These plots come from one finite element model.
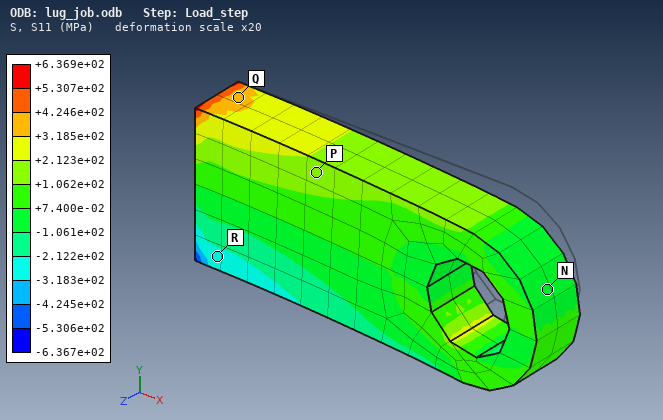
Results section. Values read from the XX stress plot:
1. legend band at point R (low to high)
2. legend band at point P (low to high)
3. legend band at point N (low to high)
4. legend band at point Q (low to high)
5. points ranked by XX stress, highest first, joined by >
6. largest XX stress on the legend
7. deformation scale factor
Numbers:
-3.183e+02 to -2.122e+02 MPa
+1.062e+02 to +2.123e+02 MPa
-1.061e+02 to +7.400e-02 MPa
+3.185e+02 to +4.246e+02 MPa
Q > P > N > R
+6.369e+02 MPa
20
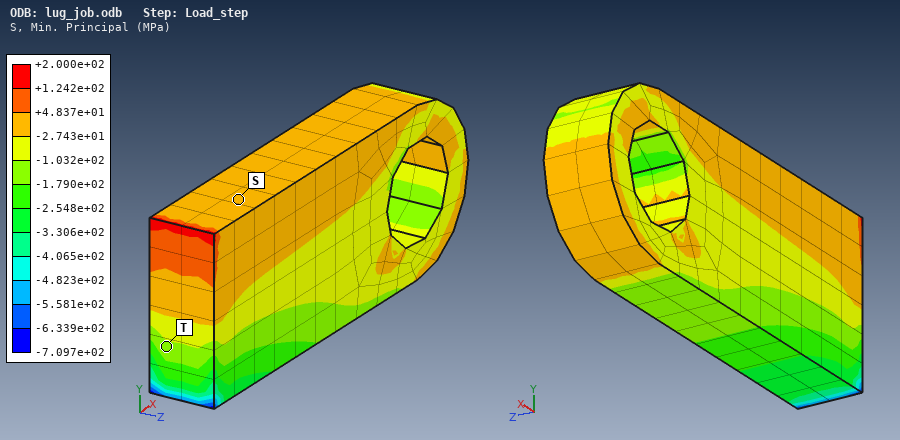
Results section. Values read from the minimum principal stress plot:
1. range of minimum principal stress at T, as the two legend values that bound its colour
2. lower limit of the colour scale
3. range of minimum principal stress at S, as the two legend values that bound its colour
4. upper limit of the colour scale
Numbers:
-1.790e+02 to -1.032e+02 MPa
-7.097e+02 MPa
-2.743e+01 to +4.837e+01 MPa
+2.000e+02 MPa
